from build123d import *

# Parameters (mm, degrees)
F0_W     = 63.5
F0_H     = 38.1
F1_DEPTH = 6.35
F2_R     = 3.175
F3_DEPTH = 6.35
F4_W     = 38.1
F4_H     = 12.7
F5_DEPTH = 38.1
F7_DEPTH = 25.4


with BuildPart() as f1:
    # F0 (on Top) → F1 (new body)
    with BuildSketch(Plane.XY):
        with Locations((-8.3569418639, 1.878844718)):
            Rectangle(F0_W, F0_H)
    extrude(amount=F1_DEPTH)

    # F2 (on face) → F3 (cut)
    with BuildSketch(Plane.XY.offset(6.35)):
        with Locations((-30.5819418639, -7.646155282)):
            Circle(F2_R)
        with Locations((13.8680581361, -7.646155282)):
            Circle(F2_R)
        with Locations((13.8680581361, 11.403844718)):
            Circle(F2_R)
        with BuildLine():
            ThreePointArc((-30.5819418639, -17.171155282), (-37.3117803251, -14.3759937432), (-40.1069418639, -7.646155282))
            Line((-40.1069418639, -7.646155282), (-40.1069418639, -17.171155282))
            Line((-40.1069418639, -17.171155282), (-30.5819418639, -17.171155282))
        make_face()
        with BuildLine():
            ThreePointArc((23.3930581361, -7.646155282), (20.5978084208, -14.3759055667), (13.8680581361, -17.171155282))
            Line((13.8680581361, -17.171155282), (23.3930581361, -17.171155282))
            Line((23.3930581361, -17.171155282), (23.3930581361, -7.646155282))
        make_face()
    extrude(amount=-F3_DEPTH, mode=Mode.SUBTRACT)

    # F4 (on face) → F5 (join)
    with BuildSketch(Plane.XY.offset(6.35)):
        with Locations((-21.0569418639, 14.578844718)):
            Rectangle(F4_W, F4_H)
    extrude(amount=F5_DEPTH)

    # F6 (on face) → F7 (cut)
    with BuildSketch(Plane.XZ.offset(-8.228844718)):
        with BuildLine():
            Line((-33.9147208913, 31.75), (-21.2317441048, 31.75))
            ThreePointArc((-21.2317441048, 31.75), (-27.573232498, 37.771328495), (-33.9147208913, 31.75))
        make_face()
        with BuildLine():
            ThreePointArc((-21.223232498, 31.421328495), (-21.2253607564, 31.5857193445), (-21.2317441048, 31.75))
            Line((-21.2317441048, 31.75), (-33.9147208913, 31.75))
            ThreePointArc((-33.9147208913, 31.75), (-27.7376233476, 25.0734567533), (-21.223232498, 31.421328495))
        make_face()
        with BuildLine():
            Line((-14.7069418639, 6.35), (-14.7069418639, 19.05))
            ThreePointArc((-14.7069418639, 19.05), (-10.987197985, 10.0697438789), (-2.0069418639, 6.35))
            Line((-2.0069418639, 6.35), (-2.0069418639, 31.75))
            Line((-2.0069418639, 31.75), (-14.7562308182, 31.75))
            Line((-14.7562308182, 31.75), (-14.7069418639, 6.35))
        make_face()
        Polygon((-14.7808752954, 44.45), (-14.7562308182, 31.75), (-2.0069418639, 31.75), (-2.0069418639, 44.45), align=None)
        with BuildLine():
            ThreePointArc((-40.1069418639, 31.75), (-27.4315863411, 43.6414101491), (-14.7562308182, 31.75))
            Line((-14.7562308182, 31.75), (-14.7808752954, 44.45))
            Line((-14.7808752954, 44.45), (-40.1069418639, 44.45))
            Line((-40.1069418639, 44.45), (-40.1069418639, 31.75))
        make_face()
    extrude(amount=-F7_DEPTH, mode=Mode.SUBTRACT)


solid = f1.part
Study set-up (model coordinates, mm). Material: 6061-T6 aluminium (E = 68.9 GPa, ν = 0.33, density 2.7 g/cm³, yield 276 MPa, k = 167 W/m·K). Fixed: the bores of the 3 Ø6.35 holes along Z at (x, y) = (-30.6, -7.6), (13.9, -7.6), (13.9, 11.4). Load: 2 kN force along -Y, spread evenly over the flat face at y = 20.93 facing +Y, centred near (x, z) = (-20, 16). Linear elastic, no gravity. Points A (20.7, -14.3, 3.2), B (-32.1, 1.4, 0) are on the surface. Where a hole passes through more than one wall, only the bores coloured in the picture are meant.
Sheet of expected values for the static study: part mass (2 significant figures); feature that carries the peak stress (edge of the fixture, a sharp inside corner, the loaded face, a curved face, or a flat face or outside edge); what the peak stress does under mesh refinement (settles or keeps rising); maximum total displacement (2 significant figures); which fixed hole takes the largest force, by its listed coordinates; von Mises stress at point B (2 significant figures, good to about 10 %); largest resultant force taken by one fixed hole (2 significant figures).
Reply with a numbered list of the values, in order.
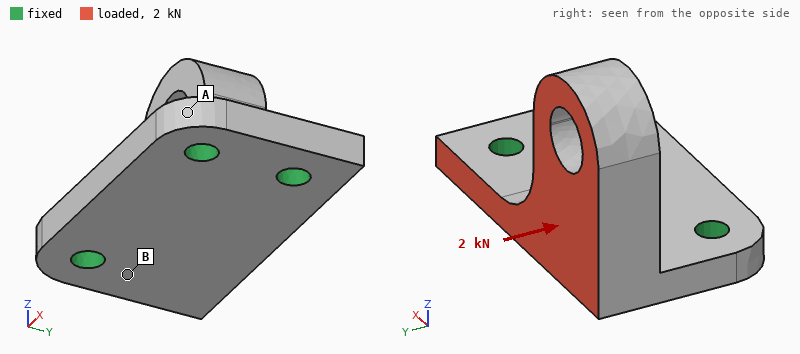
1. 66 g
2. edge of the fixture
3. keeps rising
4. 0.28 mm
5. (-30.6, -7.6)
6. 60 MPa
7. 1.4 kN
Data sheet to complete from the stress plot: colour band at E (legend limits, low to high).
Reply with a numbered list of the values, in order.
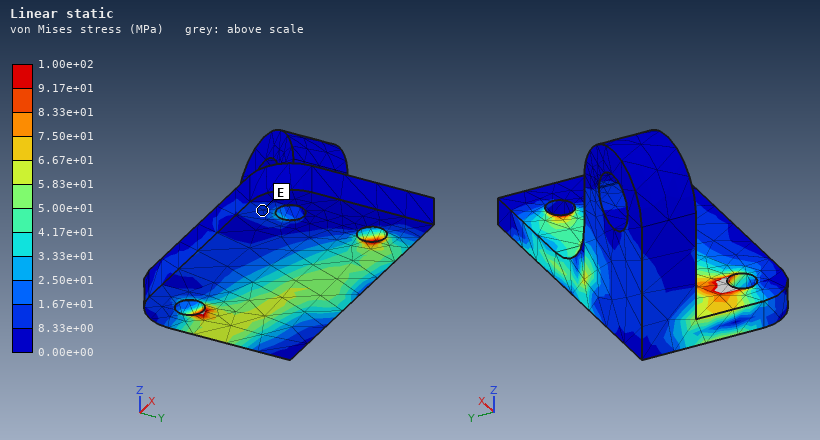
1. 8.33e+00 to 1.67e+01 MPa
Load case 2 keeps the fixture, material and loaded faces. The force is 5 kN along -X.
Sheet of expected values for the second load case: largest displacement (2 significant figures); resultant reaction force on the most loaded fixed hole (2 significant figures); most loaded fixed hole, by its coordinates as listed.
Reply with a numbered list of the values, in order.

1. 0.29 mm
2. 3.1 kN
3. (13.9, 11.4)
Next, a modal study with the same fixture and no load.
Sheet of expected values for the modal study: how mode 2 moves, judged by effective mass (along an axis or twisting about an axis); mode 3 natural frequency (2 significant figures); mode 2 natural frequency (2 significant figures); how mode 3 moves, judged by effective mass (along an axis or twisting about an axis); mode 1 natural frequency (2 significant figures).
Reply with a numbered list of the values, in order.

1. along X
2. 7500 Hz
3. 4300 Hz
4. along Z
5. 2400 Hz
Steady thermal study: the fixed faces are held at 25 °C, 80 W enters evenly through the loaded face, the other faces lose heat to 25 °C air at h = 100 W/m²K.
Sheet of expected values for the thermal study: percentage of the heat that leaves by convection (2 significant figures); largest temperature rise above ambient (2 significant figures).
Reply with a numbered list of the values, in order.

1. 17 %
2. 44 K
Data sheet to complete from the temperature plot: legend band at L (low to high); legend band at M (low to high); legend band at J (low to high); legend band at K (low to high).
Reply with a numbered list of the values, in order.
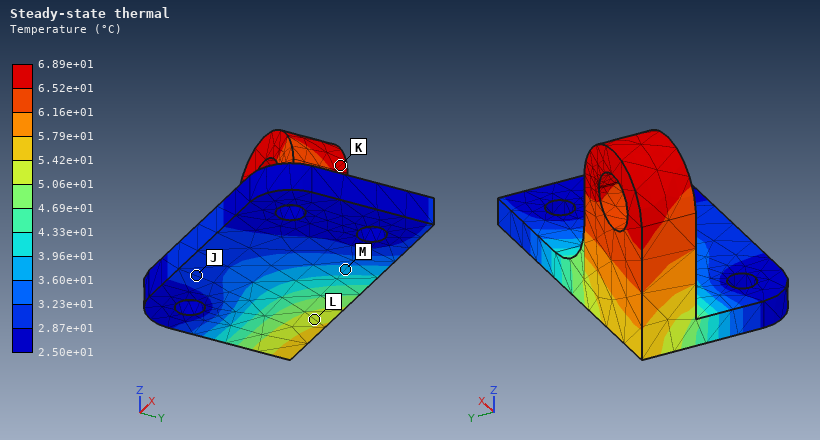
1. 5.06e+01 to 5.42e+01 °C
2. 3.60e+01 to 3.96e+01 °C
3. 2.87e+01 to 3.23e+01 °C
4. 6.52e+01 to 6.89e+01 °C
